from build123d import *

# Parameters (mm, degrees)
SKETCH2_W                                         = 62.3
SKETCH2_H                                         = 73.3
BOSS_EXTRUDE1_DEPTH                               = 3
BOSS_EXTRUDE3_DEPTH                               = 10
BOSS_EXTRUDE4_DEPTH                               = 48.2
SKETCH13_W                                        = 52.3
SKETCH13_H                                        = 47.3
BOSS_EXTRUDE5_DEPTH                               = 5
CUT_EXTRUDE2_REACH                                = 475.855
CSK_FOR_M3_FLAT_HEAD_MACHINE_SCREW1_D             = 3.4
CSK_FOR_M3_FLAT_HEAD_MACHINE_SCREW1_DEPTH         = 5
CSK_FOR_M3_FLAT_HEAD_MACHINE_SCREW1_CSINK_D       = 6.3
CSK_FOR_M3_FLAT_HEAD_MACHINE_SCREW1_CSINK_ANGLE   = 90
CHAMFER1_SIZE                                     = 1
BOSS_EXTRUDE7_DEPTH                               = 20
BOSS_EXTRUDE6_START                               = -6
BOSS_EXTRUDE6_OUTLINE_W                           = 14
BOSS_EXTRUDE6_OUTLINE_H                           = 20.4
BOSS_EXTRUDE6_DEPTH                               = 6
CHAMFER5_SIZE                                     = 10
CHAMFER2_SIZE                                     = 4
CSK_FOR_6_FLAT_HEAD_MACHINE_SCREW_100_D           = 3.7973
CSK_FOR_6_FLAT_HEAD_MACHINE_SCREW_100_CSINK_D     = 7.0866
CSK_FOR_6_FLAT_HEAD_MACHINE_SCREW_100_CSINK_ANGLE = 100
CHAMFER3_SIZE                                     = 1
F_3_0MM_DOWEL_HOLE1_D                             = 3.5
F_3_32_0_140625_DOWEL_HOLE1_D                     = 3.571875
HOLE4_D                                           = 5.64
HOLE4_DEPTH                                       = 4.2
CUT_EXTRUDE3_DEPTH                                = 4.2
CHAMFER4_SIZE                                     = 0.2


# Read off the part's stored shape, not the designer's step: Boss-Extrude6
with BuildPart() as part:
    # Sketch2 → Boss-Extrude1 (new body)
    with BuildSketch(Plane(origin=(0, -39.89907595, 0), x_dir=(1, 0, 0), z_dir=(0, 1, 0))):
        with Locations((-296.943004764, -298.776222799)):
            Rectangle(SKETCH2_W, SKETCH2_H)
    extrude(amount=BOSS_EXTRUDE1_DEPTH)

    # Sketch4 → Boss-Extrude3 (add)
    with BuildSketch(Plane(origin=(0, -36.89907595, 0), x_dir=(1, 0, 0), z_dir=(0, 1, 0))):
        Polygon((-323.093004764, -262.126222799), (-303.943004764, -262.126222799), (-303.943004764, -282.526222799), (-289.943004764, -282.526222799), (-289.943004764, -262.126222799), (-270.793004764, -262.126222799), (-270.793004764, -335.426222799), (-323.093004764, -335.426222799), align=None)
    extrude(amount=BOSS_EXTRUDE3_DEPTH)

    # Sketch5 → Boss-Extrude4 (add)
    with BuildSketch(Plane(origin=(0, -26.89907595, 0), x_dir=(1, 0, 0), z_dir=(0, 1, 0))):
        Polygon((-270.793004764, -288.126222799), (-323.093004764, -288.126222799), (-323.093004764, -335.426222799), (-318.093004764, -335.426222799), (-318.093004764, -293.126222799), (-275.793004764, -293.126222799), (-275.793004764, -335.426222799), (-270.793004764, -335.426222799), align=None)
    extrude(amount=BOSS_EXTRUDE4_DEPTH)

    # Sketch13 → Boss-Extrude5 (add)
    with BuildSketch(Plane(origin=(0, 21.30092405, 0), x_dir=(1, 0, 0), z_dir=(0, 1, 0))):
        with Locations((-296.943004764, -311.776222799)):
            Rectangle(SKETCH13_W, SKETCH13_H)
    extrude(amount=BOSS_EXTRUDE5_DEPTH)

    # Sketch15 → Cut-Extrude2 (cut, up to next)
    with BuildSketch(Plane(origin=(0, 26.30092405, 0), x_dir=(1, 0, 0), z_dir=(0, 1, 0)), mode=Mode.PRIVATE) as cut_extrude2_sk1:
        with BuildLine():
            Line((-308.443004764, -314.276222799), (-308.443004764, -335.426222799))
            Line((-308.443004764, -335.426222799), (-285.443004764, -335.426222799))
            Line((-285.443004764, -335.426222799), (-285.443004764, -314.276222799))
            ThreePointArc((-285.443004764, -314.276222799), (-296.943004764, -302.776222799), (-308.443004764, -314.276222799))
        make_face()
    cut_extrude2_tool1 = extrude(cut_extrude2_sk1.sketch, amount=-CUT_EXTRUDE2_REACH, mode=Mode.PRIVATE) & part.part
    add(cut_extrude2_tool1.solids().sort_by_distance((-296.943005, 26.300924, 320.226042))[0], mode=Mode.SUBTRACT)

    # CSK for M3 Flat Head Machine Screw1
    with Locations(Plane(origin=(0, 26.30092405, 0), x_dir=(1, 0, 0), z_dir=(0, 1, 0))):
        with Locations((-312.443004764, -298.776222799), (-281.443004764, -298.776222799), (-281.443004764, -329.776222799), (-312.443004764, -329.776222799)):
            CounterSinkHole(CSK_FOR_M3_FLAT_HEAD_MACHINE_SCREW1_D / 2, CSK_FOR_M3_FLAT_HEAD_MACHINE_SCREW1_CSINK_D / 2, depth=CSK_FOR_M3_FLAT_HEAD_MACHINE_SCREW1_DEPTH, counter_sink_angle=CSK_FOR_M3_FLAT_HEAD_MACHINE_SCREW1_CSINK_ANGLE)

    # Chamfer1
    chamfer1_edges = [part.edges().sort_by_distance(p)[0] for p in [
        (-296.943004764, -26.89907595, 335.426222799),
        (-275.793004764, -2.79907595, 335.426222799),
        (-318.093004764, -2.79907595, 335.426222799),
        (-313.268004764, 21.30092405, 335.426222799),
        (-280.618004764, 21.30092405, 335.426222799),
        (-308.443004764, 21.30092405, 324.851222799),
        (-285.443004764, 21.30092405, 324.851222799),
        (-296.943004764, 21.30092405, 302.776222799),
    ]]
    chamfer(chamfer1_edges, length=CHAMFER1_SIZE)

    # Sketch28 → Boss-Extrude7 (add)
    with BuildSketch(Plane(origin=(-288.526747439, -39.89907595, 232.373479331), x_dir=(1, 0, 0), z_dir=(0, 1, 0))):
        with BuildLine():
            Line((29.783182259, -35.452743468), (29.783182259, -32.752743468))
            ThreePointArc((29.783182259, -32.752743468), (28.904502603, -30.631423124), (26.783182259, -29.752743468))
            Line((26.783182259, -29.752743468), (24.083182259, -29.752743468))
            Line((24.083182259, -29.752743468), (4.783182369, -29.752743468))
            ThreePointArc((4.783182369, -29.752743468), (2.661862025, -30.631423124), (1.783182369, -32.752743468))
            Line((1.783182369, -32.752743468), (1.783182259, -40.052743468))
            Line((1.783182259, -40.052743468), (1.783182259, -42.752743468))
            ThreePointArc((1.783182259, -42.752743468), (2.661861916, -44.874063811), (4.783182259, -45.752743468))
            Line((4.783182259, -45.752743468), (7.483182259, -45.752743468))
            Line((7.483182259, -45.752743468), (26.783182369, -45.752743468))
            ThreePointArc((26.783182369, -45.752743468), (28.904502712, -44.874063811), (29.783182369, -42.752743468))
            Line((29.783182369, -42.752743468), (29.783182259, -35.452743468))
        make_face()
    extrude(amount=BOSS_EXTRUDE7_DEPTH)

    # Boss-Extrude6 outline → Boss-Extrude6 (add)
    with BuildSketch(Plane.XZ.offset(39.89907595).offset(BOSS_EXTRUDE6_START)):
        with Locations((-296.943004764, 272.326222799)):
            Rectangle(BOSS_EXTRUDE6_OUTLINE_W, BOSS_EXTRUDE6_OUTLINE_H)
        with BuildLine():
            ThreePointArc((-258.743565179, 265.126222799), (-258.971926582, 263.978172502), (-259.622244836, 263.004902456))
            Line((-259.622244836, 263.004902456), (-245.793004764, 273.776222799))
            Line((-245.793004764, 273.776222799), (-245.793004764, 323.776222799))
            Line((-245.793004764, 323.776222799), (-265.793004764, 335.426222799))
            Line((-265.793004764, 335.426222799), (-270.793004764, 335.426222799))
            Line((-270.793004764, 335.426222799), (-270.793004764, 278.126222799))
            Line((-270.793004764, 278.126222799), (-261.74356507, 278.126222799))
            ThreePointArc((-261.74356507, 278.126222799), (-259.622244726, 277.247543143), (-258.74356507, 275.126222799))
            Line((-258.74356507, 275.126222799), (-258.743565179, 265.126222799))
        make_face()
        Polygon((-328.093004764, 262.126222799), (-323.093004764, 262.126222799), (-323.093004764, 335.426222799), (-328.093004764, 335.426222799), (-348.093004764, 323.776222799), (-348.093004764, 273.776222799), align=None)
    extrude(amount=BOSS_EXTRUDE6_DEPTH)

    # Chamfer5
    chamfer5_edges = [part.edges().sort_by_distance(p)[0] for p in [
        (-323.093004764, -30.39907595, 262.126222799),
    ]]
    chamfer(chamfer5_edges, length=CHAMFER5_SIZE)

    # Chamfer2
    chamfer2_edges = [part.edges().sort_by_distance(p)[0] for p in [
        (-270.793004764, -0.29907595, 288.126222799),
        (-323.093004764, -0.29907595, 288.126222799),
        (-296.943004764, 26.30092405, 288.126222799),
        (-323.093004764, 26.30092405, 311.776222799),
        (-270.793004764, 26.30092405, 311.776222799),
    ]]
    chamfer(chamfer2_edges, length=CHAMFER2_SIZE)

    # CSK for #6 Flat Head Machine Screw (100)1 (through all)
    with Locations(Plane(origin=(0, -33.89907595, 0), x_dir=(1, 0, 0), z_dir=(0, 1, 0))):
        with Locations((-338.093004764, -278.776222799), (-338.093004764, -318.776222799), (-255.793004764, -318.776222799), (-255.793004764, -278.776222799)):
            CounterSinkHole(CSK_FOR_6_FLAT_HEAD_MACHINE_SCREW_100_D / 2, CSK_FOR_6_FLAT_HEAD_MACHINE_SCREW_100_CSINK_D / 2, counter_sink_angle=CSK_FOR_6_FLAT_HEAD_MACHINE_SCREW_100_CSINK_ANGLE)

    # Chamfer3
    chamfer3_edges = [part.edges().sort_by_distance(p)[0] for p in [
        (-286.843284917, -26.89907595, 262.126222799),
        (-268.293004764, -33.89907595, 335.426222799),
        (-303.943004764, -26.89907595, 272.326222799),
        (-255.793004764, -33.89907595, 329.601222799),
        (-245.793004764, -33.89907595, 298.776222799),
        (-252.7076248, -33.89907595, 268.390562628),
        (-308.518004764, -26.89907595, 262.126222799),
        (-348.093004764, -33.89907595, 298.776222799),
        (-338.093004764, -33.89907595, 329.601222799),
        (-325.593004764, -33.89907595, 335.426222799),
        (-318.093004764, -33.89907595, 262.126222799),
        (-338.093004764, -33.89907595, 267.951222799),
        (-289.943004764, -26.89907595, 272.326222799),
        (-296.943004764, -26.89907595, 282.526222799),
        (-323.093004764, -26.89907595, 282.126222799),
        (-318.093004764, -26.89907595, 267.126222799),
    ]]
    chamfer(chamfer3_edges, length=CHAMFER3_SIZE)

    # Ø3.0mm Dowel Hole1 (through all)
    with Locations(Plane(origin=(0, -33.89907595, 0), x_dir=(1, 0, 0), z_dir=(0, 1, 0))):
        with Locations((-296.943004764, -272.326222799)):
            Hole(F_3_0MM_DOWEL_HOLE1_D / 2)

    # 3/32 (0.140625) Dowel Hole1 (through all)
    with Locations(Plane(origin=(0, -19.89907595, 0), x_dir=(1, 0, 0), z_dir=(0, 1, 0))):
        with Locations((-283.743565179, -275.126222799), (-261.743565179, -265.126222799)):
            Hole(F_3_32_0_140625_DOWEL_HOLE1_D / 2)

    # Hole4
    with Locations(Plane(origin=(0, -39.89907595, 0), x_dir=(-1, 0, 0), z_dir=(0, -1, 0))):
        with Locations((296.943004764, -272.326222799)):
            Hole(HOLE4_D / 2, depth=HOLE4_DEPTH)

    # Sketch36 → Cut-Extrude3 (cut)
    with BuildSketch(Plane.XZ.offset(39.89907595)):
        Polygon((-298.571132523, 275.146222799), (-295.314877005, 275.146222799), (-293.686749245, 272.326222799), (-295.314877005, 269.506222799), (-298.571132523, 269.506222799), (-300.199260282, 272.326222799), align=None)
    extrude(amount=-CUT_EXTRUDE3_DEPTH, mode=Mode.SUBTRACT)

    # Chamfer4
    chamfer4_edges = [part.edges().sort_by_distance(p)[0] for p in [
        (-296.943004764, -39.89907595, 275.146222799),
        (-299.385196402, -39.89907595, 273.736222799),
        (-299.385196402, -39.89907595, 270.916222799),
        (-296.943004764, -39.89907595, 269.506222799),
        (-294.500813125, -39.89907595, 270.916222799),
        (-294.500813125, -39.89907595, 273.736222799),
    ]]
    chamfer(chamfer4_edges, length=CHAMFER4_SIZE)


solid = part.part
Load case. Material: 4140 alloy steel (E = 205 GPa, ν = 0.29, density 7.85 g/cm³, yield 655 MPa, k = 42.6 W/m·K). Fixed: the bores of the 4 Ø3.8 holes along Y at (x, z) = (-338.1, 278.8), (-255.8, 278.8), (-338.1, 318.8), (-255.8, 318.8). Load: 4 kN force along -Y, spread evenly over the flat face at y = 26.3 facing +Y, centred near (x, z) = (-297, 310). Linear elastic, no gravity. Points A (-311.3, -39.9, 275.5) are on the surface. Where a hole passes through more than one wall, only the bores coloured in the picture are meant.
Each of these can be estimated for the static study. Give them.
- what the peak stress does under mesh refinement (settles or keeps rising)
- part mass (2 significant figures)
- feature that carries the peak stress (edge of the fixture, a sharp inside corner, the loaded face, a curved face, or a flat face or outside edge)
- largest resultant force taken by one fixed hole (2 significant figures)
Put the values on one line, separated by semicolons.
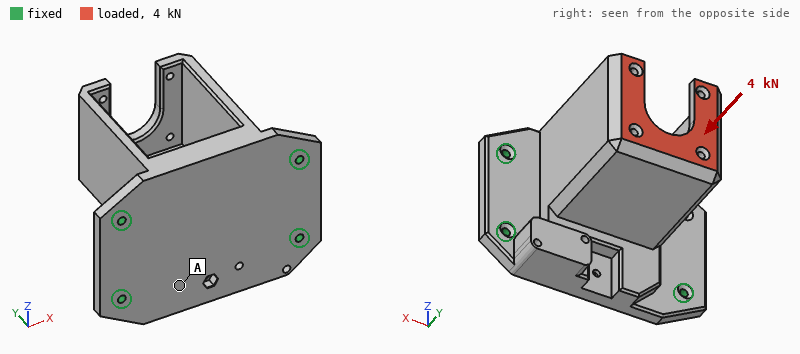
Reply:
keeps rising; 860 g; edge of the fixture; 1.8 kN
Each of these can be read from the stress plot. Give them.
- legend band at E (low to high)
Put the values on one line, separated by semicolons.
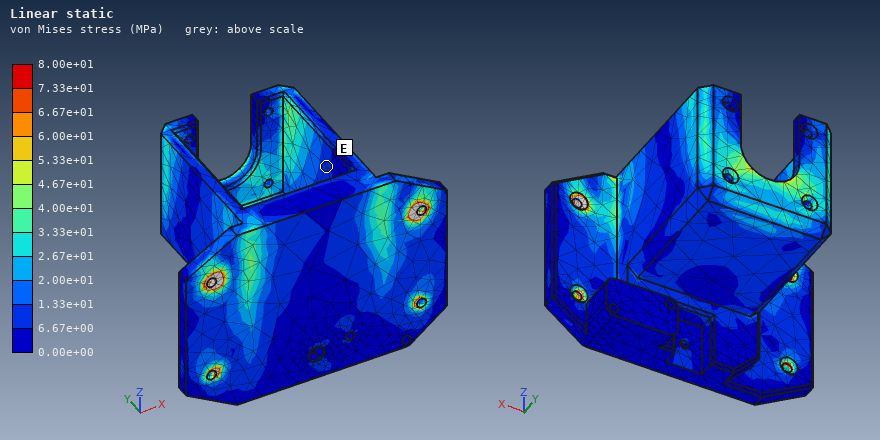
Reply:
6.67e+00 to 1.33e+01 MPa
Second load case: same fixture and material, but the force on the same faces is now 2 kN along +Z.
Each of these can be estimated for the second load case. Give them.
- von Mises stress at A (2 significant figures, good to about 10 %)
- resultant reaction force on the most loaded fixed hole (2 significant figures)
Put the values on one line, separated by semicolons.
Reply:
16 MPa; 1.9 kN
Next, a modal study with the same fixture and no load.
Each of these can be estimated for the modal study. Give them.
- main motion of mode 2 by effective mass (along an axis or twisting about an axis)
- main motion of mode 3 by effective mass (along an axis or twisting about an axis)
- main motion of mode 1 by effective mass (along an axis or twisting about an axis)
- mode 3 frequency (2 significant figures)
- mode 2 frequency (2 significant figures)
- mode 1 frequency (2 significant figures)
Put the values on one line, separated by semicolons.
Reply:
along X; along Y; along Z; 3600 Hz; 2700 Hz; 2300 Hz
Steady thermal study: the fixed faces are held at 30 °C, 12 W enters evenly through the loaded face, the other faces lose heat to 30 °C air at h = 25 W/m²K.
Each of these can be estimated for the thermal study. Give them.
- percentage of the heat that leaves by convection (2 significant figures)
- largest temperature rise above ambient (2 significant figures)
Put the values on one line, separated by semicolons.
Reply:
55 %; 23 K
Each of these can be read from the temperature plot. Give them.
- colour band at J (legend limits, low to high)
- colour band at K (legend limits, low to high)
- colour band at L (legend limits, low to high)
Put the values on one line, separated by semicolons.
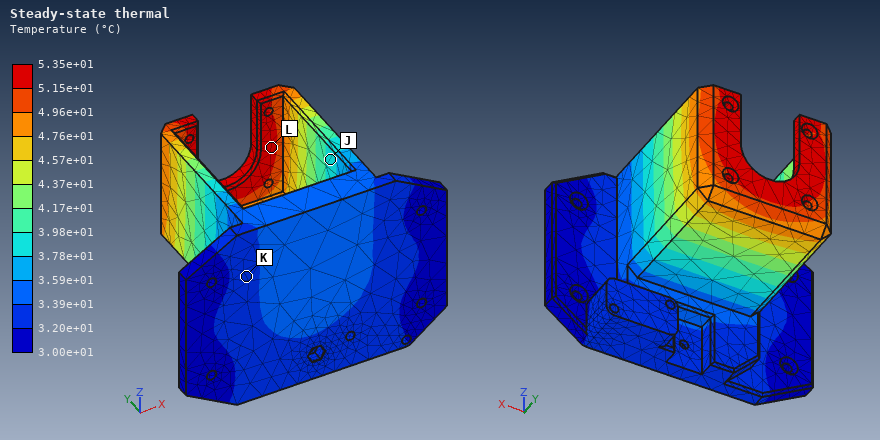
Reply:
3.78e+01 to 3.98e+01 °C; 3.20e+01 to 3.39e+01 °C; 5.15e+01 to 5.35e+01 °C
